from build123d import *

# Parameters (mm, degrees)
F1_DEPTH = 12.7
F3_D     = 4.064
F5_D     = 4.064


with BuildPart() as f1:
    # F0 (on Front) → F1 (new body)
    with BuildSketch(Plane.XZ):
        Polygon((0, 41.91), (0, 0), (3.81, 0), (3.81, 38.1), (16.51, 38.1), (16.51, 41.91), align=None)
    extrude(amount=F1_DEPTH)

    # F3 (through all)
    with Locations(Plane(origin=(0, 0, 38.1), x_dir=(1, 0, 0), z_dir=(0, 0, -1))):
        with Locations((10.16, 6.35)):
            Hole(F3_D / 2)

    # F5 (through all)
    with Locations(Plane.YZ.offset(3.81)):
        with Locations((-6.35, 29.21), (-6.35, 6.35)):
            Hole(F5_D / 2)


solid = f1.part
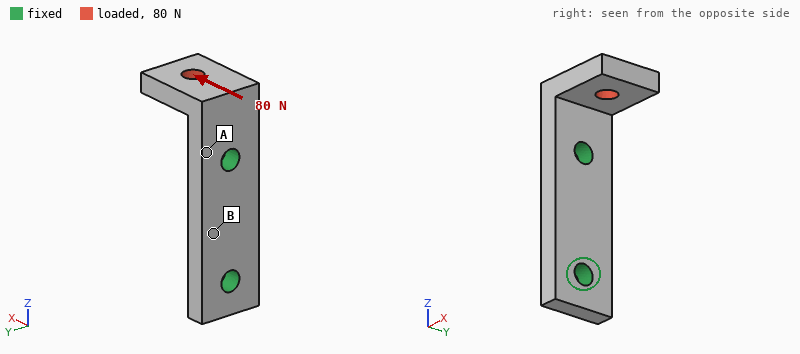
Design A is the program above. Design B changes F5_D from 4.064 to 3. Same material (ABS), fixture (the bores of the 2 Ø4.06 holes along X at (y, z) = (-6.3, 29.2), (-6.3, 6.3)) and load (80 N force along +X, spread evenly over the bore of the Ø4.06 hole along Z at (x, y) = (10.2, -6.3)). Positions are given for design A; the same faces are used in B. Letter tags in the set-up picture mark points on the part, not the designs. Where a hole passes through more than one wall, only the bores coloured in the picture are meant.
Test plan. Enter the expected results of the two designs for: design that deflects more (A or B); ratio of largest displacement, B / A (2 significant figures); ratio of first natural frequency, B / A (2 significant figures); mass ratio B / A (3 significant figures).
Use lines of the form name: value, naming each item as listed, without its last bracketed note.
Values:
design that deflects more: B
ratio of largest displacement, B / A: 1.2
ratio of first natural frequency, B / A: 0.95
mass ratio B / A: 1.02
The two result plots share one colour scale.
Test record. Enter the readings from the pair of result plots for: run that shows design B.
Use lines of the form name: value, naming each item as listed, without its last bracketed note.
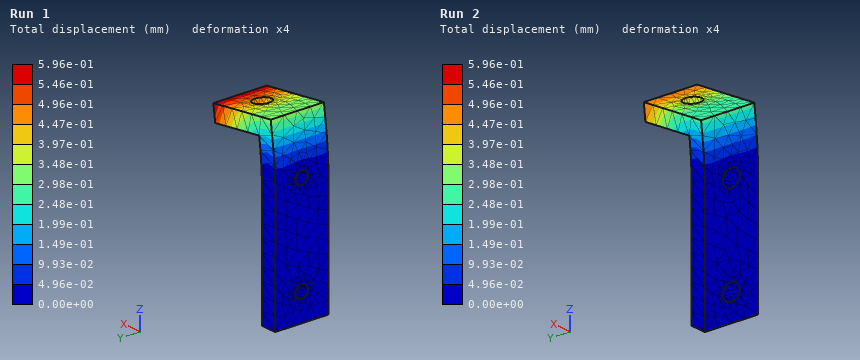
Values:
run that shows design B: Run 1
